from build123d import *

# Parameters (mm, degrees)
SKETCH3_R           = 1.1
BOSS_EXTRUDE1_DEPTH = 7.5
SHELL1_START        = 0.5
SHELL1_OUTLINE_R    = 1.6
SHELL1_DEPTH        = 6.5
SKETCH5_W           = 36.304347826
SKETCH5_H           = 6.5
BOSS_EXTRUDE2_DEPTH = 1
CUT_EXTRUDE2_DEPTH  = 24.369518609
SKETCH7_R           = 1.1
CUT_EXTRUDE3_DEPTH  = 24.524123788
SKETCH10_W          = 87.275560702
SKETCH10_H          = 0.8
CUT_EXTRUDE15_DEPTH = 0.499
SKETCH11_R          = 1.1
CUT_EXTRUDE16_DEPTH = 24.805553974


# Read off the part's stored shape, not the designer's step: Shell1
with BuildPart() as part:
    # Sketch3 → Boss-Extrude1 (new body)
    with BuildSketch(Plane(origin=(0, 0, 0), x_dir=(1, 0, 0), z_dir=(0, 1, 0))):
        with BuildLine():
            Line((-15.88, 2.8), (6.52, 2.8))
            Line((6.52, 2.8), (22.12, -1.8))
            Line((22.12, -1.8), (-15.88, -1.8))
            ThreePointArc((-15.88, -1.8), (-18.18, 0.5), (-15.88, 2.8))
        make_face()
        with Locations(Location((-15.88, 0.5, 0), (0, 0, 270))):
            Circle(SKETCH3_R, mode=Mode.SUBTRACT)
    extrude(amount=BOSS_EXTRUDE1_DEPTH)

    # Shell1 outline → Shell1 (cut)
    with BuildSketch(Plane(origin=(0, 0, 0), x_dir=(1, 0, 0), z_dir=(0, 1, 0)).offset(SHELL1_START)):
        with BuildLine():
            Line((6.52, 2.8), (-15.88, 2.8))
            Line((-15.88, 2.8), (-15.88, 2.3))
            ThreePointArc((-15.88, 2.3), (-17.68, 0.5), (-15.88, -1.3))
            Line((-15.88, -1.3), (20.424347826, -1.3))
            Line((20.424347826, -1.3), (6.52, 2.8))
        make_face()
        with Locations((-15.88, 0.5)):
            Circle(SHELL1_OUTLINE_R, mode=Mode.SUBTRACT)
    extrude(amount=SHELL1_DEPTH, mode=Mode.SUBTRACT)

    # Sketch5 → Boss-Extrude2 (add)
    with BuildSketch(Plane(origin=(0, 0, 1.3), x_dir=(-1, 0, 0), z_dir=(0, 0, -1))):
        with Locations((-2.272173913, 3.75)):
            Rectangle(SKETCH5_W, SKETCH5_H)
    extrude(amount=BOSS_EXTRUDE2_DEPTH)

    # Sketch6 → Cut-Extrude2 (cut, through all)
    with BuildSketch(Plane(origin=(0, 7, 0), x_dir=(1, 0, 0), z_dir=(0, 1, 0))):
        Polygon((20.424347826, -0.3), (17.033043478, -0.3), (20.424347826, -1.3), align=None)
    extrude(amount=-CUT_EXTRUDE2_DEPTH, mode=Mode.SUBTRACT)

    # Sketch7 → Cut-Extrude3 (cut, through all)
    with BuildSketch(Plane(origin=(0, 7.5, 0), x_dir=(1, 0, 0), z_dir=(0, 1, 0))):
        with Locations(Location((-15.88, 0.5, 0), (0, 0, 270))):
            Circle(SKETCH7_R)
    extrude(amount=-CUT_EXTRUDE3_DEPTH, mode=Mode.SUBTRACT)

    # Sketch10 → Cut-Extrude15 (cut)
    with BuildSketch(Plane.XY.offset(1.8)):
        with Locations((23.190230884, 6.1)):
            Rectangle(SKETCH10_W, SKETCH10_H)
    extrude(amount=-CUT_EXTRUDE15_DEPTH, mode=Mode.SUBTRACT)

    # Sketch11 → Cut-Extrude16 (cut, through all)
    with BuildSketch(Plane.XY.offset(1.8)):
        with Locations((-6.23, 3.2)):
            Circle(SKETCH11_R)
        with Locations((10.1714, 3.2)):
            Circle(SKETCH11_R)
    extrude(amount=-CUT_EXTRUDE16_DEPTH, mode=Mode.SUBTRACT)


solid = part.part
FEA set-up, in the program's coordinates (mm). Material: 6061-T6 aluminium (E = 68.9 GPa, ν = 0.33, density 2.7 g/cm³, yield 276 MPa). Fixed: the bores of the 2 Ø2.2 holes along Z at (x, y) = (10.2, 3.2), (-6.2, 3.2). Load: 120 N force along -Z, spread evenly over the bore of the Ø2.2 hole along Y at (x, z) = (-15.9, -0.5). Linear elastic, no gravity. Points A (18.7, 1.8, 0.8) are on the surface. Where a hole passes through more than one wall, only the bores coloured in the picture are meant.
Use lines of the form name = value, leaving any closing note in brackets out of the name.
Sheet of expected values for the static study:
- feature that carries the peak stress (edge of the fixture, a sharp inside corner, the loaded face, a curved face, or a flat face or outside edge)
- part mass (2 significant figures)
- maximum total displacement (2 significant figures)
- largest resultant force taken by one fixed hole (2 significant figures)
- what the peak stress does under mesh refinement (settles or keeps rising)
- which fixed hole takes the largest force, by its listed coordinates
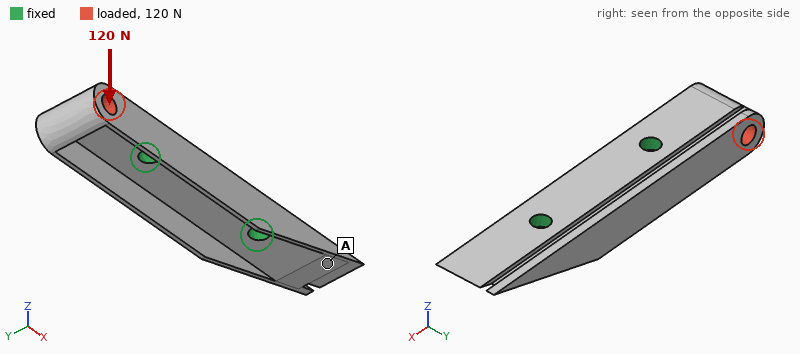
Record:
feature that carries the peak stress = edge of the fixture
part mass = 1.4 g
maximum total displacement = 86 µm
largest resultant force taken by one fixed hole = 180 N
what the peak stress does under mesh refinement = keeps rising
which fixed hole takes the largest force, by its listed coordinates = (-6.2, 3.2)
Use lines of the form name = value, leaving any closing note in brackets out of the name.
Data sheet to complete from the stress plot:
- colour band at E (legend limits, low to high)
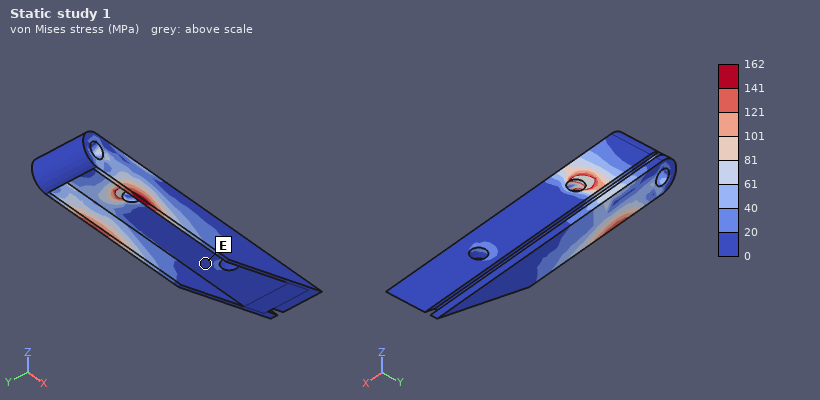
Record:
colour band at E = 0 to 20 MPa
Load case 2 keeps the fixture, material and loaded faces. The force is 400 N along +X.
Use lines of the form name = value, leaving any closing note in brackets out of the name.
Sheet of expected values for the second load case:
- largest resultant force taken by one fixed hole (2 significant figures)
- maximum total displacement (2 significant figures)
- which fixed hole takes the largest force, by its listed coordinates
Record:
largest resultant force taken by one fixed hole = 320 N
maximum total displacement = 46 µm
which fixed hole takes the largest force, by its listed coordinates = (-6.2, 3.2)
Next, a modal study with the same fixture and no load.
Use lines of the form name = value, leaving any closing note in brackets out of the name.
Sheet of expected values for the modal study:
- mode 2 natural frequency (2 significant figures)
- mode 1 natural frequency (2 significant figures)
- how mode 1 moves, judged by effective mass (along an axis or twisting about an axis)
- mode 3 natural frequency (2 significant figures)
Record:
mode 2 natural frequency = 18 kHz
mode 1 natural frequency = 13 kHz
how mode 1 moves, judged by effective mass = along Z
mode 3 natural frequency = 18 kHz
